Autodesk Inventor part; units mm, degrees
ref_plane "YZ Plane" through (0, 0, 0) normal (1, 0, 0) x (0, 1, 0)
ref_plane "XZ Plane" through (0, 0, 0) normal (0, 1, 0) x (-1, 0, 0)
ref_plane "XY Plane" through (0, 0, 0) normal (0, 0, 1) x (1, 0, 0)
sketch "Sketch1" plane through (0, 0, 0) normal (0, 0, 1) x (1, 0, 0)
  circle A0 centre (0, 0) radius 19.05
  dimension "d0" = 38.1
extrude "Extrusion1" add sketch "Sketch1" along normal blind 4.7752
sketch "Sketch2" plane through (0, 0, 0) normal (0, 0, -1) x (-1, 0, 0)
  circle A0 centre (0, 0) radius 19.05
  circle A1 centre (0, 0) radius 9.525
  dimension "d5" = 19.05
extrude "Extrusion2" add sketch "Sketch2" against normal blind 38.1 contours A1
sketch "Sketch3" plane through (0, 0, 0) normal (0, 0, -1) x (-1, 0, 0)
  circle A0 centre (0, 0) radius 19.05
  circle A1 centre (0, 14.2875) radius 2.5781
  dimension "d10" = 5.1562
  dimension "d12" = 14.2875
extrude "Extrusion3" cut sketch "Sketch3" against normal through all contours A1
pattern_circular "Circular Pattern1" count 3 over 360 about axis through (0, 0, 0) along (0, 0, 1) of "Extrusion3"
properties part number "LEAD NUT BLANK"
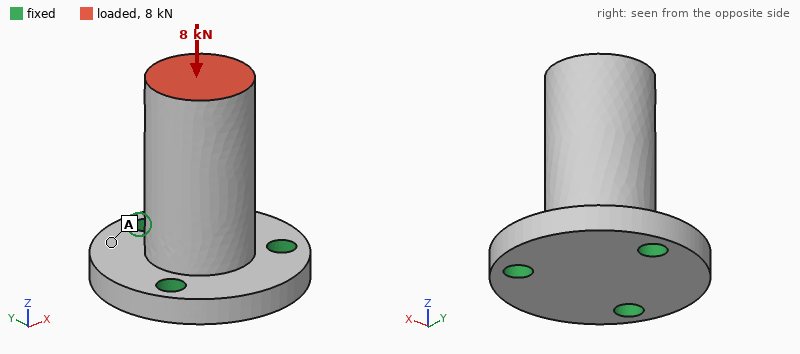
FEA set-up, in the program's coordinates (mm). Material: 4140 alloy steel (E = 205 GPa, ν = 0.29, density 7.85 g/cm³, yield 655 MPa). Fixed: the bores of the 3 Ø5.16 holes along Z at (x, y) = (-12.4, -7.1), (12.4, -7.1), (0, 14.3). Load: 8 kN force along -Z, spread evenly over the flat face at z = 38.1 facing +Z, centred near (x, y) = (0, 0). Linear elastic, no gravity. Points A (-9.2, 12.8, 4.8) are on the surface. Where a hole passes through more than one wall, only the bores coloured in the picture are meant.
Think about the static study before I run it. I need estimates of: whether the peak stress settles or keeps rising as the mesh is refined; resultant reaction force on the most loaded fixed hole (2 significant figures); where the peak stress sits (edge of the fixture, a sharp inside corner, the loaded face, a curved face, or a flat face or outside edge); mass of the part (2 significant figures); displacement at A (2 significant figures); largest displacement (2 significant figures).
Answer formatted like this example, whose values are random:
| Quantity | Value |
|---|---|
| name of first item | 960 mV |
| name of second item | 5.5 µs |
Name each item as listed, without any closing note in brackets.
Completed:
| Quantity | Value |
|---|---|
| whether the peak stress settles or keeps rising as the mesh is refined | keeps rising |
| resultant reaction force on the most loaded fixed hole | 2.8 kN |
| where the peak stress sits | edge of the fixture |
| mass of the part | 110 g |
| displacement at A | 2.3 µm |
| largest displacement | 9.6 µm |
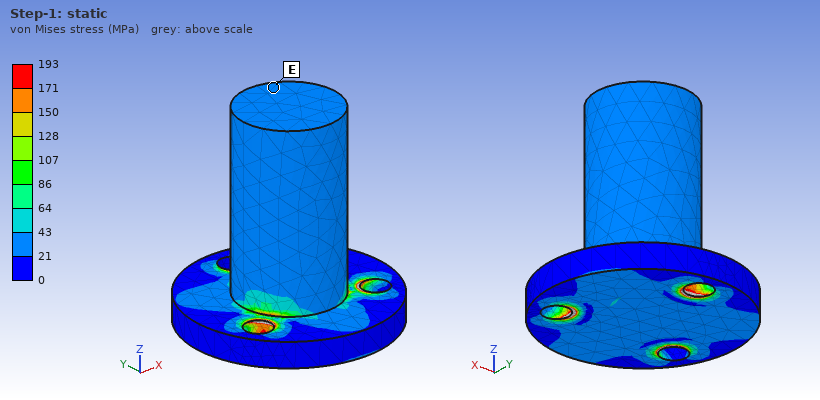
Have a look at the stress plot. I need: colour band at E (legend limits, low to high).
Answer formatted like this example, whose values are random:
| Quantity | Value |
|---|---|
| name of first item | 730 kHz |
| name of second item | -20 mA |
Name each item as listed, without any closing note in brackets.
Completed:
| Quantity | Value |
|---|---|
| colour band at E | 21 to 43 MPa |
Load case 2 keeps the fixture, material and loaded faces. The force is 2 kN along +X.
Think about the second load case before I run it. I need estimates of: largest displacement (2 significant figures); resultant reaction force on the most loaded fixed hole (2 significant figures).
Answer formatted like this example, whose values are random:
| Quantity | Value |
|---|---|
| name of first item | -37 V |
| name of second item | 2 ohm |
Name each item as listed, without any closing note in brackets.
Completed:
| Quantity | Value |
|---|---|
| largest displacement | 48 µm |
| resultant reaction force on the most loaded fixed hole | 3.2 kN |
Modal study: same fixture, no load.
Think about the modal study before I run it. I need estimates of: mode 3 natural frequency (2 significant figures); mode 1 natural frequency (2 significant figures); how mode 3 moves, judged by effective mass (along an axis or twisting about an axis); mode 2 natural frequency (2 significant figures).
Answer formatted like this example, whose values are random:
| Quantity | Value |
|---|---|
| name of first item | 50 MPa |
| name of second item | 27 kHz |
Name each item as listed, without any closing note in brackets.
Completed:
| Quantity | Value |
|---|---|
| mode 3 natural frequency | 19 kHz |
| mode 1 natural frequency | 6800 Hz |
| how mode 3 moves, judged by effective mass | along Z |
| mode 2 natural frequency | 6800 Hz |
